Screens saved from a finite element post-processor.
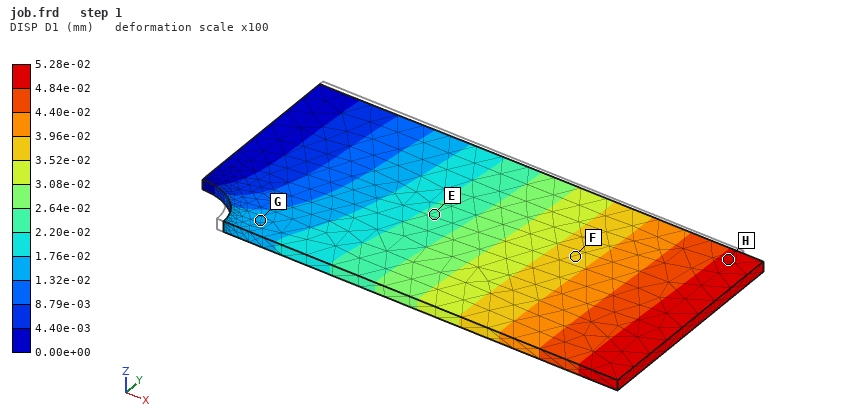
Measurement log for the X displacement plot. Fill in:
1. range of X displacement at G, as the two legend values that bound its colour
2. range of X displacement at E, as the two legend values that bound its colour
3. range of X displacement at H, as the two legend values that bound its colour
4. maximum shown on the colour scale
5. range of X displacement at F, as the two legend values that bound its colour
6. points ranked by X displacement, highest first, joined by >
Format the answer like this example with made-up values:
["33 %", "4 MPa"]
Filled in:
["1.32e-02 to 1.76e-02 mm", "2.20e-02 to 2.64e-02 mm", "4.84e-02 to 5.28e-02 mm", "5.28e-02 mm", "3.52e-02 to 3.96e-02 mm", "H > F > E > G"]
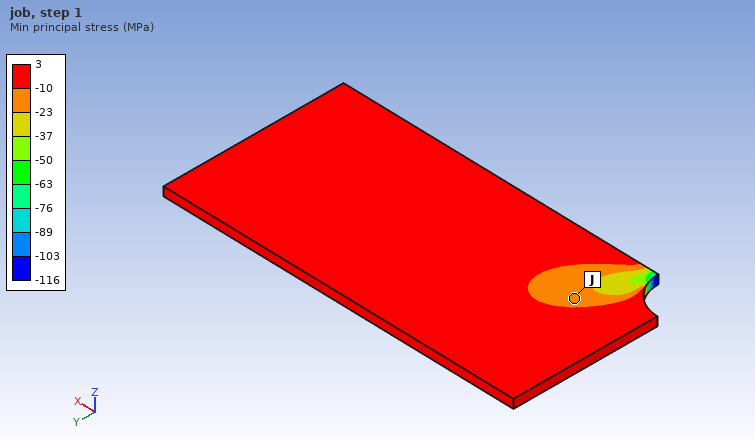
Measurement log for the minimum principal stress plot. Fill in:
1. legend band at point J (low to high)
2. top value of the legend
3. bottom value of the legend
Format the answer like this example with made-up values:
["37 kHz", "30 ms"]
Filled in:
["-23 to -10 MPa", "3 MPa", "-116 MPa"]
